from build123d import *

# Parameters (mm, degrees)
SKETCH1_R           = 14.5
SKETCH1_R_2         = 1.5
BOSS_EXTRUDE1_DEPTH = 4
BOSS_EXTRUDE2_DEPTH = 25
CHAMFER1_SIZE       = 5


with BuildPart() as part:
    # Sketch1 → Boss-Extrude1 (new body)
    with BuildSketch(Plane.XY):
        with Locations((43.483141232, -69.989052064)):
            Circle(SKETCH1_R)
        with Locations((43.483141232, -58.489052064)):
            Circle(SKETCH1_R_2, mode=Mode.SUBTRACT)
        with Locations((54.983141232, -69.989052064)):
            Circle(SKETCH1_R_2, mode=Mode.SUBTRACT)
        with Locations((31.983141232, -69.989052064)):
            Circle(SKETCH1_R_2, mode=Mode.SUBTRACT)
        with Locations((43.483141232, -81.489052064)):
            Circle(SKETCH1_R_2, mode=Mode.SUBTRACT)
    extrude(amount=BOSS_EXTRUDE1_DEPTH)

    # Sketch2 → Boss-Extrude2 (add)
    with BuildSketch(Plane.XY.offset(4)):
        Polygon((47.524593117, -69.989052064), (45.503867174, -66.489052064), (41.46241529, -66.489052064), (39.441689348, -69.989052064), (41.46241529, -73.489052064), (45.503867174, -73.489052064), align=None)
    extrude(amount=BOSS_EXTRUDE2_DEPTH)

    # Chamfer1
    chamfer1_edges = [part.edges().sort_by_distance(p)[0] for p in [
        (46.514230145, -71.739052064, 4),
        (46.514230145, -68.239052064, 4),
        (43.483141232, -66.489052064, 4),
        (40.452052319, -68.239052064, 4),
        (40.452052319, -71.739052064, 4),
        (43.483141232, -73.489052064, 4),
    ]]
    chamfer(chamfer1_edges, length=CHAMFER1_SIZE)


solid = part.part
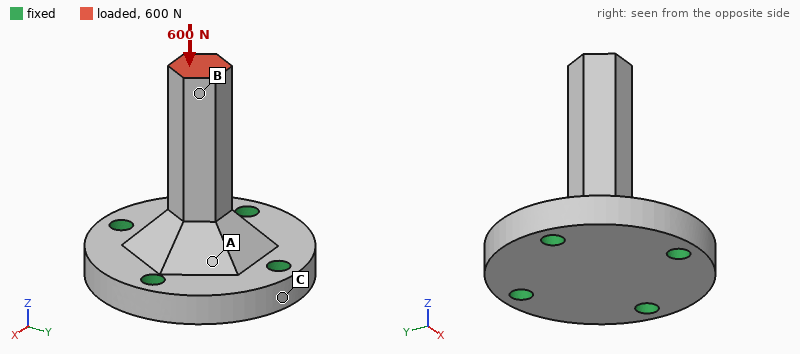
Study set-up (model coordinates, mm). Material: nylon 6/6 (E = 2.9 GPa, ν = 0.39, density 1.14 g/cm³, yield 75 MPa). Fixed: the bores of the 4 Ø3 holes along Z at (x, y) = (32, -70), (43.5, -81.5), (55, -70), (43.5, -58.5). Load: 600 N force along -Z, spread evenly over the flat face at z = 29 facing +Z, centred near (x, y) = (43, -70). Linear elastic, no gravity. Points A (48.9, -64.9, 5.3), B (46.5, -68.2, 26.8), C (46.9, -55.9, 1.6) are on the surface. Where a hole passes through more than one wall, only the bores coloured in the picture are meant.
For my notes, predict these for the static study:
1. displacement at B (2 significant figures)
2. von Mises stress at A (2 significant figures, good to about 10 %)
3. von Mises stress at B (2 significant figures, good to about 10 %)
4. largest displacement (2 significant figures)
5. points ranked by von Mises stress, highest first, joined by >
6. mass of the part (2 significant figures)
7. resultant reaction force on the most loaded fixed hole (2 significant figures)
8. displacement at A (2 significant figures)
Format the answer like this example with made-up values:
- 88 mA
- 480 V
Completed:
- 0.13 mm
- 5.4 MPa
- 14 MPa
- 0.14 mm
- B > A > C
- 4.6 g
- 170 N
- 0.025 mm
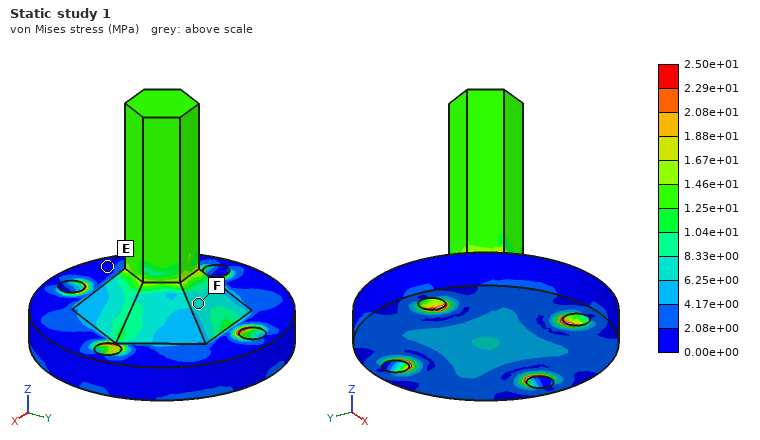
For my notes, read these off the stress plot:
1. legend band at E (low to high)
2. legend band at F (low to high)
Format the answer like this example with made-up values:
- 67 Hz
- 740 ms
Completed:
- 0.00e+00 to 2.08e+00 MPa
- 6.25e+00 to 8.33e+00 MPa
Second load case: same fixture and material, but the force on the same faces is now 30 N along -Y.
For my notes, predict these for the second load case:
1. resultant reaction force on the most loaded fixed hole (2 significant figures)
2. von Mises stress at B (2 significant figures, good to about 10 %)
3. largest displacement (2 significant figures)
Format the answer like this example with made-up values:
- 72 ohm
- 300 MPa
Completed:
- 40 N
- 1.8 MPa
- 0.29 mm
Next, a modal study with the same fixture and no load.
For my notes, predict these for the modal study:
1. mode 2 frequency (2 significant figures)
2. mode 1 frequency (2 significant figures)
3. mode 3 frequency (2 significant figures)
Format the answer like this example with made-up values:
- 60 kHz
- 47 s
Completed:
- 3100 Hz
- 3100 Hz
- 11 kHz
